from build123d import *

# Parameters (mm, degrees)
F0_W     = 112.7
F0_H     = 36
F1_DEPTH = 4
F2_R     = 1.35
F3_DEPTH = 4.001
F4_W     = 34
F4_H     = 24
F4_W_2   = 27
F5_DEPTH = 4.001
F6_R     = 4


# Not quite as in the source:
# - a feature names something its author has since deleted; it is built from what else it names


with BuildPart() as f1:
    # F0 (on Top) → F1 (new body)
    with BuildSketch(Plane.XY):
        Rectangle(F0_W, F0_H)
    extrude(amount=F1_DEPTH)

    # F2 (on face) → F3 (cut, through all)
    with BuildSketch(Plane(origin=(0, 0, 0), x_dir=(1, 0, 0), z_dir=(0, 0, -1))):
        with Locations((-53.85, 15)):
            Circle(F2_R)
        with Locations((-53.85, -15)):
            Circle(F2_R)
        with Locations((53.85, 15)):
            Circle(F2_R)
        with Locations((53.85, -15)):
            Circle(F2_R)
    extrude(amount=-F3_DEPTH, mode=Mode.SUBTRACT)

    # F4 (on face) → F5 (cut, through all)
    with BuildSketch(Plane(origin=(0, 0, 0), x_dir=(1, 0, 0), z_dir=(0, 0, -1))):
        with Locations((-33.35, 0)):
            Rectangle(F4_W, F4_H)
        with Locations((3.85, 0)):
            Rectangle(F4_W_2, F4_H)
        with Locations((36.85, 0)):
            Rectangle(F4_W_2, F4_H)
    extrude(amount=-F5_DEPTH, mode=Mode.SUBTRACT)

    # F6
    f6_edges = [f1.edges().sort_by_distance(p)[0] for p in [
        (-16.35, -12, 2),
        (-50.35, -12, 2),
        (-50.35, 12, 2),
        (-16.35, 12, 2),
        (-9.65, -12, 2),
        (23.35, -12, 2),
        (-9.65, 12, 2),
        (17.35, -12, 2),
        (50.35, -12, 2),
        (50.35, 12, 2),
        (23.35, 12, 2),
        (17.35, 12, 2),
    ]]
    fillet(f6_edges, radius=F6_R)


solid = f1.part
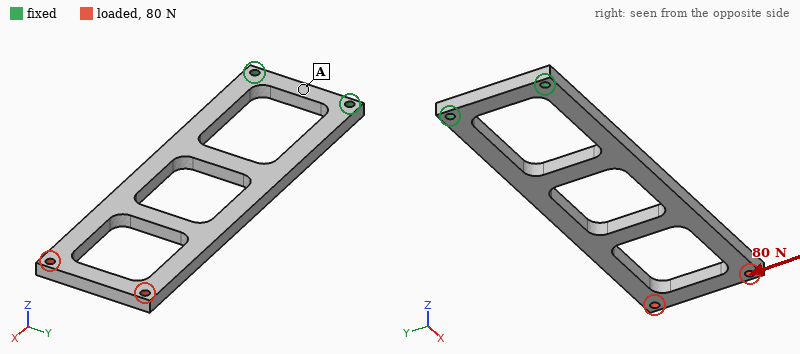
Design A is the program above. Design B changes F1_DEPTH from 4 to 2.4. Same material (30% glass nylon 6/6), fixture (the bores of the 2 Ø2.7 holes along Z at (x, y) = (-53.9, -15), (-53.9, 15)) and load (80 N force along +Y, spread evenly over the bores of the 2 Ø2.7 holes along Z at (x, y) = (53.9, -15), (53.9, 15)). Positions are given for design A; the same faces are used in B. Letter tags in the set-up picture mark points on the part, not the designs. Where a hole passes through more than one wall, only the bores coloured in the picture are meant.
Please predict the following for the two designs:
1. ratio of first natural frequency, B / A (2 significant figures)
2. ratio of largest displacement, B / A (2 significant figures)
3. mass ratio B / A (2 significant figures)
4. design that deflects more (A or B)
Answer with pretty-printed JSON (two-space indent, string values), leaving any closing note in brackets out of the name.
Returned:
{
  "ratio of first natural frequency, B / A": "0.60",
  "ratio of largest displacement, B / A": "1.7",
  "mass ratio B / A": "0.60",
  "design that deflects more": "B"
}
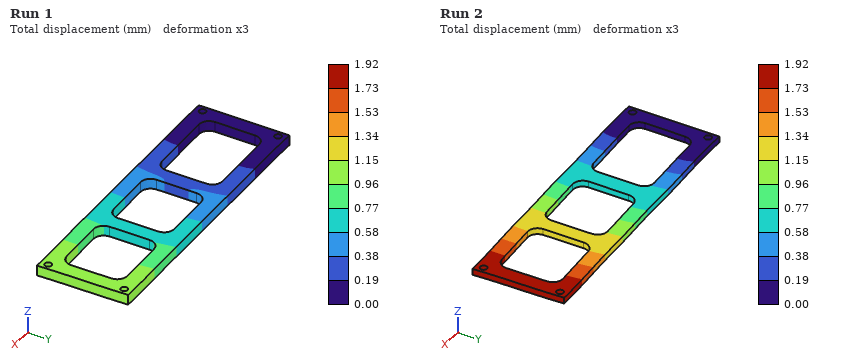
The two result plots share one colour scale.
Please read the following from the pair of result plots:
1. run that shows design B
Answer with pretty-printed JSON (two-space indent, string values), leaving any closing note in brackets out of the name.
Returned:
{
  "run that shows design B": "Run 2"
}
